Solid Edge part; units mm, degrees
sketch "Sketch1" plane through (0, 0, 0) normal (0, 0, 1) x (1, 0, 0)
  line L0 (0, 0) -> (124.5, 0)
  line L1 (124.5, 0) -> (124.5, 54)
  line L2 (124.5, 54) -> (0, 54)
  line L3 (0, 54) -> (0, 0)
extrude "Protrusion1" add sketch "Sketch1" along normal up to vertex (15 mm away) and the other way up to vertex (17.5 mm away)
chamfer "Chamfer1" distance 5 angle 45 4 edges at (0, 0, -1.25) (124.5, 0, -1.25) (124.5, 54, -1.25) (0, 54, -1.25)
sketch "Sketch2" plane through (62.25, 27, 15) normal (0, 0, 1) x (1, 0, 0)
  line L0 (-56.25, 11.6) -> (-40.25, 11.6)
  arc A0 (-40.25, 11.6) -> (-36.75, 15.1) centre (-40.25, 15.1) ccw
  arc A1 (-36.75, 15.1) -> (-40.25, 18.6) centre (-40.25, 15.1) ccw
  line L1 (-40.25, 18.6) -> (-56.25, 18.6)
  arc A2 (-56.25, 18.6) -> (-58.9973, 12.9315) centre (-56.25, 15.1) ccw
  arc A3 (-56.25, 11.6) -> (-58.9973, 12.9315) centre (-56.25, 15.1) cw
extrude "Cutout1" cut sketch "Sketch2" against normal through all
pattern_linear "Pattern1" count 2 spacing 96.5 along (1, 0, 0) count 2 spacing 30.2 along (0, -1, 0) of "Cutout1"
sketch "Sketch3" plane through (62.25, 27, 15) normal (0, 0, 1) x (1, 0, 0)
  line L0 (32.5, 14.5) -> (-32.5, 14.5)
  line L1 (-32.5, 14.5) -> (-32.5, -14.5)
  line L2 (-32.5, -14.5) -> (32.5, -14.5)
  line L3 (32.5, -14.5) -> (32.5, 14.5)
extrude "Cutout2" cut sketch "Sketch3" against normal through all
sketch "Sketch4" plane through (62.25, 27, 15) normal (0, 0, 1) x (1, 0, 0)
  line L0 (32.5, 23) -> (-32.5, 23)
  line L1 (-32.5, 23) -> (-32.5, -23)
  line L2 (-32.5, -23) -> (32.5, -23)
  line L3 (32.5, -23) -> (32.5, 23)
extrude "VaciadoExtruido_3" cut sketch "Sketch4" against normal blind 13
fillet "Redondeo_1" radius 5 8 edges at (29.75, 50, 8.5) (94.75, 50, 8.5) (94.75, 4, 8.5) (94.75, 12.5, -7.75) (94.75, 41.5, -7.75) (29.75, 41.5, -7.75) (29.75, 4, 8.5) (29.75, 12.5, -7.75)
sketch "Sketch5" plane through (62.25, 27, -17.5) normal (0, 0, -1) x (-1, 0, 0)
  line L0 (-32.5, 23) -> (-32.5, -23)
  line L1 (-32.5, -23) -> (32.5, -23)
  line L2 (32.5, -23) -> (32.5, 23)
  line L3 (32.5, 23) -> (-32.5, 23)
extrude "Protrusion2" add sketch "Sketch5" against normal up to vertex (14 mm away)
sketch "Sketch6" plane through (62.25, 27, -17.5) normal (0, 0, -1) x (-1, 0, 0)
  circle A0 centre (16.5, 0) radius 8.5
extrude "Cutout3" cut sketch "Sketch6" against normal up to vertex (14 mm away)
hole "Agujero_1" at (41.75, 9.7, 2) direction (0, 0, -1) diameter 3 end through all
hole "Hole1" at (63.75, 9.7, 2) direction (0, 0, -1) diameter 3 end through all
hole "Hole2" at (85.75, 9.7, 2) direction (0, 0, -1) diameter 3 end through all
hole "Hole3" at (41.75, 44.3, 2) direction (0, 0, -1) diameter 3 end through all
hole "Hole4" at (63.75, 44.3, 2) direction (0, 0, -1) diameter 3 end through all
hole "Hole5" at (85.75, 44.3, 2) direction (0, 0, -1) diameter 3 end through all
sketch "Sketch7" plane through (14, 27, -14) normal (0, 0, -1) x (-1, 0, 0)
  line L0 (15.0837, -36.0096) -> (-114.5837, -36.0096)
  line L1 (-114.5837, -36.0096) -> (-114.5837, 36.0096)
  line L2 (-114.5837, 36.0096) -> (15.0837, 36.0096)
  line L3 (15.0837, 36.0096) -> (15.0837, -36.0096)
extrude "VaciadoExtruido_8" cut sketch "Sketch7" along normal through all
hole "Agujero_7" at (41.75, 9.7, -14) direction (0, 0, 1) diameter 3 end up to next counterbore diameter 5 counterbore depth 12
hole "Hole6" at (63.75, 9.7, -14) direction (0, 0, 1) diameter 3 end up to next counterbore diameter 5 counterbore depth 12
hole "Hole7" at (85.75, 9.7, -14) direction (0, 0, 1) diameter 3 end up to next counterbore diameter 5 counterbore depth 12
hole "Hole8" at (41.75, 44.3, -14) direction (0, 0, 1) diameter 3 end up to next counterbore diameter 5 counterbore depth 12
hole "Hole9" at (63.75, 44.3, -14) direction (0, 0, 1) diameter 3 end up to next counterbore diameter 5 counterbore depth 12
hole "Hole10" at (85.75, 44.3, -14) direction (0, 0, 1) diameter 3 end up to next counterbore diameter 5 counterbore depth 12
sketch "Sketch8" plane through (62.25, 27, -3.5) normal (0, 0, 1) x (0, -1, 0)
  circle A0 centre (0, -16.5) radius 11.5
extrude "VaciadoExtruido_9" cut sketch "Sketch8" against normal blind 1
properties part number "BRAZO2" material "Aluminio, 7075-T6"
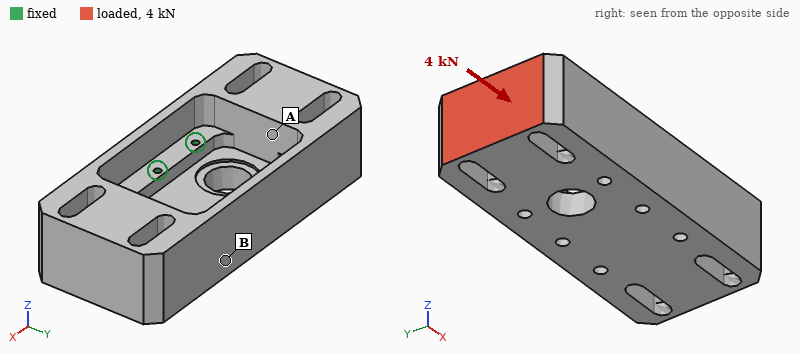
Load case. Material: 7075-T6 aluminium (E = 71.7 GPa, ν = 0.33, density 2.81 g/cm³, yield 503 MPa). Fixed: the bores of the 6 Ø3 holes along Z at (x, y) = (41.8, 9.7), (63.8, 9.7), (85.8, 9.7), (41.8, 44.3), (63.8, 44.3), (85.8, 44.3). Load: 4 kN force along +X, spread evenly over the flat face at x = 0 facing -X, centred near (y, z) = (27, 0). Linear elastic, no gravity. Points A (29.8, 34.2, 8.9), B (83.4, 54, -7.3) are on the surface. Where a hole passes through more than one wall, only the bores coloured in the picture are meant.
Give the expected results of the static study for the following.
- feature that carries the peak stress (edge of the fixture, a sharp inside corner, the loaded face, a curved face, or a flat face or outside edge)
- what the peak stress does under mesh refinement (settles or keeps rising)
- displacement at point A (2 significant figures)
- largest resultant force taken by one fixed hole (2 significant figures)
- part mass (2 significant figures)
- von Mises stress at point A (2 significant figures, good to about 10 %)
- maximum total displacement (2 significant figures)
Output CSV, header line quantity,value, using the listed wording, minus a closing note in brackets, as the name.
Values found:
quantity,value
feature that carries the peak stress,edge of the fixture
what the peak stress does under mesh refinement,keeps rising
displacement at point A,9.6 µm
largest resultant force taken by one fixed hole,1.2 kN
part mass,350 g
von Mises stress at point A,7.3 MPa
maximum total displacement,17 µm
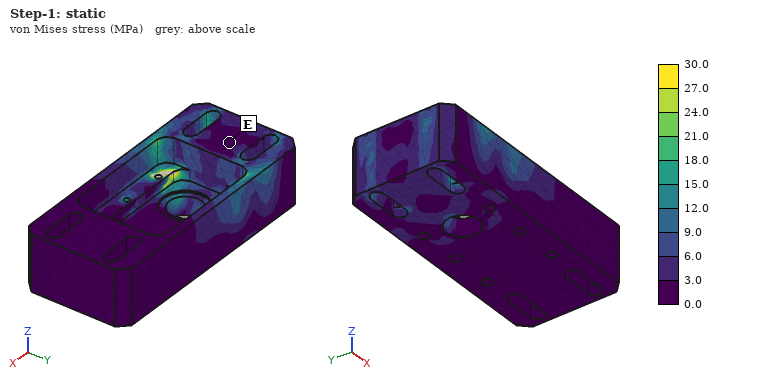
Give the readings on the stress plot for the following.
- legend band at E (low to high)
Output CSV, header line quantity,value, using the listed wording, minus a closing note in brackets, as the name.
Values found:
quantity,value
legend band at E,0.0 to 3.0 MPa
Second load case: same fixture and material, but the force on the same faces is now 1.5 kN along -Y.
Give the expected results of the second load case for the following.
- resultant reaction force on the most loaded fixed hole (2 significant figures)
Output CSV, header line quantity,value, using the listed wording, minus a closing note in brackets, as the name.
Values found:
quantity,value
resultant reaction force on the most loaded fixed hole,1.1 kN
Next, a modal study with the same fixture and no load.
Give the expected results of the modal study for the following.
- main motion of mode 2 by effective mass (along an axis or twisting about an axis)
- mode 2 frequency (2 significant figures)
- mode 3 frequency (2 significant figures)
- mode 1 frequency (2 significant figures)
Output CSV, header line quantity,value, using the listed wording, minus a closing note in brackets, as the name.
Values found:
quantity,value
main motion of mode 2 by effective mass,along Z
mode 2 frequency,4600 Hz
mode 3 frequency,6200 Hz
mode 1 frequency,3800 Hz
